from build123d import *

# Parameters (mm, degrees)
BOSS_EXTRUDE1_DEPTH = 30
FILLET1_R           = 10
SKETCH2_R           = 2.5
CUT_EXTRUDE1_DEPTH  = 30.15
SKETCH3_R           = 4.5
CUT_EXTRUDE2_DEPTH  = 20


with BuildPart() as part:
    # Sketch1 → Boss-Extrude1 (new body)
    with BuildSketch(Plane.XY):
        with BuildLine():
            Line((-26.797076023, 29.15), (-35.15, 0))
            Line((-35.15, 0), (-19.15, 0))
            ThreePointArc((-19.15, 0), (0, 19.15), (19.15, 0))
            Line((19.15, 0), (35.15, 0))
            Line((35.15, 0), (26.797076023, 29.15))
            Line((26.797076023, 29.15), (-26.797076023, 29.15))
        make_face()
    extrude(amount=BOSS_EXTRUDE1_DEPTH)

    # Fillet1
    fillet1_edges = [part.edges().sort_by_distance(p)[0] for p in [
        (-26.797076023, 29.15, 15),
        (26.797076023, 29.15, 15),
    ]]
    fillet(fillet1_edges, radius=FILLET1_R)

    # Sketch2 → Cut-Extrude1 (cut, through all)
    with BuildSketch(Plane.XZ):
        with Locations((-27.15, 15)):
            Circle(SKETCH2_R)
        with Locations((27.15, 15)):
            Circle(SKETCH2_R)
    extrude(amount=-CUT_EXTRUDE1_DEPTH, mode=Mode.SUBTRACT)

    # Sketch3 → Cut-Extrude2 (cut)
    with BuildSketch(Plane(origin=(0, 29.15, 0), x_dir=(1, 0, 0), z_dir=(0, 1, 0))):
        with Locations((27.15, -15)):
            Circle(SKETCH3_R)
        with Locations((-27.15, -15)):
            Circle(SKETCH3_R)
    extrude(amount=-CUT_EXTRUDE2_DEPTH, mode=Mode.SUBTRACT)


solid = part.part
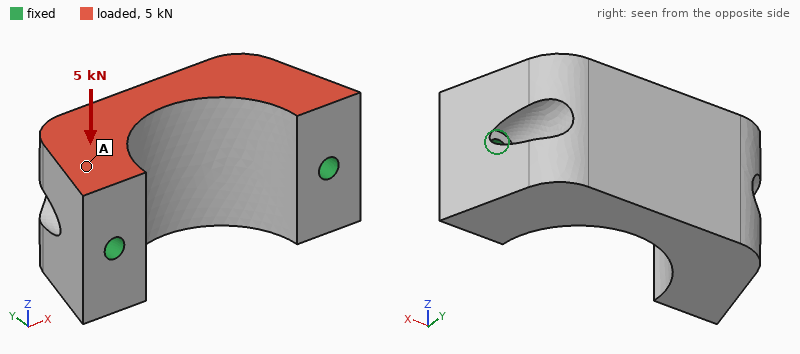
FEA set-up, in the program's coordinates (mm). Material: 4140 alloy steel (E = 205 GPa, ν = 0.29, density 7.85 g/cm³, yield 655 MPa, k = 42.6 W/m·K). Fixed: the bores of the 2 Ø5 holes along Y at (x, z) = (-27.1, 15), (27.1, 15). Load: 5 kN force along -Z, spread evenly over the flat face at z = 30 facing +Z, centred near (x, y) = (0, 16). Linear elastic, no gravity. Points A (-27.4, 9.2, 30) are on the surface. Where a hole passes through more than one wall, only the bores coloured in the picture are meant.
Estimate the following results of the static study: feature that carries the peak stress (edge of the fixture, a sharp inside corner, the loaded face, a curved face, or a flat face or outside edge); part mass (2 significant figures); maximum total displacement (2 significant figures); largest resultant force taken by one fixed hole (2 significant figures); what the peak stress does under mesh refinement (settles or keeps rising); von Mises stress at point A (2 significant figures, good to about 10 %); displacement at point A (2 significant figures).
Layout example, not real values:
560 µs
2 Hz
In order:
edge of the fixture
270 g
16 µm
2.5 kN
keeps rising
15 MPa
6.9 µm
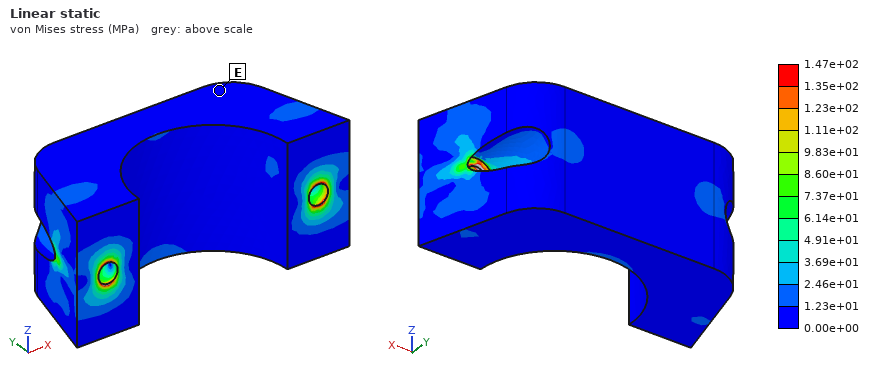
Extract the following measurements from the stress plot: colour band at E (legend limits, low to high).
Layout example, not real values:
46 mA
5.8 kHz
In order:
0.00e+00 to 1.23e+01 MPa
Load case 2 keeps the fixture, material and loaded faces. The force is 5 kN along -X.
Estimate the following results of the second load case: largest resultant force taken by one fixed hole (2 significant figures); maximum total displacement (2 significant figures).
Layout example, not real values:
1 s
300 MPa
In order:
2.8 kN
7.7 µm
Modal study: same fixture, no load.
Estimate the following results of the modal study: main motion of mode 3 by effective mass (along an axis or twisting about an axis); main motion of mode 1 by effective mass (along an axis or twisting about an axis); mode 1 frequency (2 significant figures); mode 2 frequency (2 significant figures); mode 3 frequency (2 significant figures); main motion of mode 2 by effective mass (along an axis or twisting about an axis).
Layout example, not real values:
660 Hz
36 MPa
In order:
along X
along Z
6200 Hz
13 kHz
14 kHz
twisting about Y
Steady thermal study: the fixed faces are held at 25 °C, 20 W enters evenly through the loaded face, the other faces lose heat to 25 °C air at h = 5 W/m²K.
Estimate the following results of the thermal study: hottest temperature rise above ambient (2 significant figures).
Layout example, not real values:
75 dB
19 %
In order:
17 K
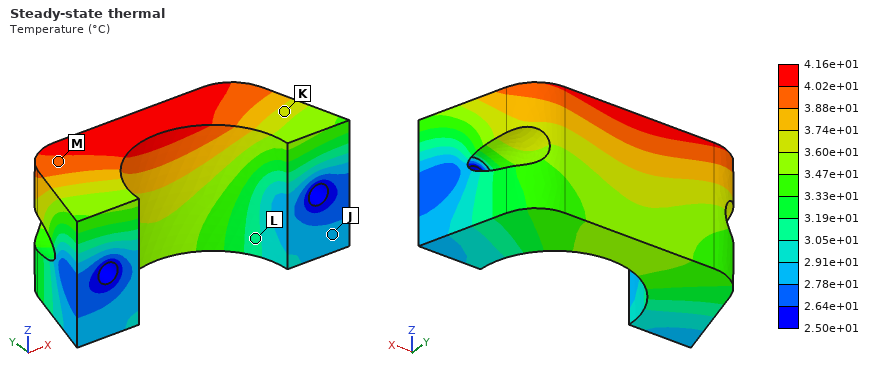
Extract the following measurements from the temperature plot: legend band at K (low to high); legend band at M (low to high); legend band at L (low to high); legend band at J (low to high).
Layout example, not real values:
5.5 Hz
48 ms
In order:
3.60e+01 to 3.74e+01 °C
3.88e+01 to 4.02e+01 °C
3.05e+01 to 3.19e+01 °C
2.78e+01 to 2.91e+01 °C
